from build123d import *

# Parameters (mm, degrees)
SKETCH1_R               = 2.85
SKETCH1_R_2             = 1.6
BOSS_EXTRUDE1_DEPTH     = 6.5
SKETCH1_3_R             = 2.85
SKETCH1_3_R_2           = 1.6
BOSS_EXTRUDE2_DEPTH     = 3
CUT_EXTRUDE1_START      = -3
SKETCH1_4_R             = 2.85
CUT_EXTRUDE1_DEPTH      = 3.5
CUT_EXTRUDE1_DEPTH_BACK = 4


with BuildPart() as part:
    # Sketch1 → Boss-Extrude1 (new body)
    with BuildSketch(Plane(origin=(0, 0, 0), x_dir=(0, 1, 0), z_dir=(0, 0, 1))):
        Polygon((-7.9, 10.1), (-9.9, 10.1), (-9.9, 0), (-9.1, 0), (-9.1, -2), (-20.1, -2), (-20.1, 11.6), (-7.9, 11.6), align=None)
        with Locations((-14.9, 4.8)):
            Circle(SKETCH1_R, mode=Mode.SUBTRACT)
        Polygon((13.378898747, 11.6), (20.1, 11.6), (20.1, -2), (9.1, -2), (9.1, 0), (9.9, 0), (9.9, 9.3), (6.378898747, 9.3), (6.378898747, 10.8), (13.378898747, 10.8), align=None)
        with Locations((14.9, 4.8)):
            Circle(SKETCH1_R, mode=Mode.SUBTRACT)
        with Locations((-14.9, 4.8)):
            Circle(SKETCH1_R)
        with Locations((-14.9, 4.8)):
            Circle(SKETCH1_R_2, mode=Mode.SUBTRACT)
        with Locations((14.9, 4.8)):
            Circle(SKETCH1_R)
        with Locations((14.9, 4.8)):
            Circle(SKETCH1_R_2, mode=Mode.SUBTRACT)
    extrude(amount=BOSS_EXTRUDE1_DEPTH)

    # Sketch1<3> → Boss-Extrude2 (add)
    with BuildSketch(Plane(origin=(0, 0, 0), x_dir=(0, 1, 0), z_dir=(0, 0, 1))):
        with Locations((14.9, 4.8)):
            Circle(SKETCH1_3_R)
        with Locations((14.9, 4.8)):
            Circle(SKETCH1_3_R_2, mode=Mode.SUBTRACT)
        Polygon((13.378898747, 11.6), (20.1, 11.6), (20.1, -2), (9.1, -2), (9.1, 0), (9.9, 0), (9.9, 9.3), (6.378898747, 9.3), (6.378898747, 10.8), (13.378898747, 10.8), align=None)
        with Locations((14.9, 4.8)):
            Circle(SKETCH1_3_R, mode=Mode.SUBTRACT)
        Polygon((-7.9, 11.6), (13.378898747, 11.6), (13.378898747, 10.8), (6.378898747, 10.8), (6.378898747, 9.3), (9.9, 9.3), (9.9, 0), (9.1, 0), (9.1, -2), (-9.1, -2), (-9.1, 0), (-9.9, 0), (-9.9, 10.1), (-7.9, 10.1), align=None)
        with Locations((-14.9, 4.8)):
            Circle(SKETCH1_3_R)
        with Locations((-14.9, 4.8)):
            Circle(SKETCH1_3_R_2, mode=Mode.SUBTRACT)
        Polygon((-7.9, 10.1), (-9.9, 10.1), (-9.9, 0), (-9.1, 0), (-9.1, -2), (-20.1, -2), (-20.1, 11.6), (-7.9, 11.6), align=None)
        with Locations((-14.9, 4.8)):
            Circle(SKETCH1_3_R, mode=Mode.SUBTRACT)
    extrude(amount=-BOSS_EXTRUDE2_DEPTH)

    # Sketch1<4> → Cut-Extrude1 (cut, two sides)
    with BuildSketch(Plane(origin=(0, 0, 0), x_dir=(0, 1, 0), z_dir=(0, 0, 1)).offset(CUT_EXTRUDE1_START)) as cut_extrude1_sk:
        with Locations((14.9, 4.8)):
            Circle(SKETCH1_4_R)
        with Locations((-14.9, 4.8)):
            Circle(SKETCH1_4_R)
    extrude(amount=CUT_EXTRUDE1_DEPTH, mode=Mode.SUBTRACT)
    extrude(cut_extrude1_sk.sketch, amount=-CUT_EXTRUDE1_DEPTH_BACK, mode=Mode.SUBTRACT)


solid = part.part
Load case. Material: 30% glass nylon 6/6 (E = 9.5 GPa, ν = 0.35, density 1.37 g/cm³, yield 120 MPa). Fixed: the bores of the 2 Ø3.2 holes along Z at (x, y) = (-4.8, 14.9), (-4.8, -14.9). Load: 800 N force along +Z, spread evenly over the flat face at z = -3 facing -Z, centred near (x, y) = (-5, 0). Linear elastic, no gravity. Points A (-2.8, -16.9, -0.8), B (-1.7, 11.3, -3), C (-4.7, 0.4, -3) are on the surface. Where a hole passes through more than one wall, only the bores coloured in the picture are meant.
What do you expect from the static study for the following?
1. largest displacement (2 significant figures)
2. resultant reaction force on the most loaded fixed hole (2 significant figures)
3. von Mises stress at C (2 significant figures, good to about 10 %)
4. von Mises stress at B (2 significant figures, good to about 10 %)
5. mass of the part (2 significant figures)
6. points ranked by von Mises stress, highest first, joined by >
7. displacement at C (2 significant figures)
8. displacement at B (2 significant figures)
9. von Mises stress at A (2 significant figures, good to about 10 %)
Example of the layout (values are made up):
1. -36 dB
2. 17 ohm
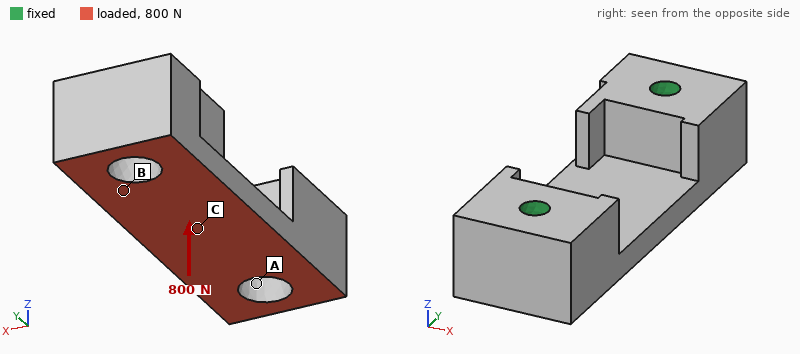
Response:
1. 72 µm
2. 450 N
3. 22 MPa
4. 12 MPa
5. 4.4 g
6. C > B > A
7. 60 µm
8. 13 µm
9. 4.5 MPa
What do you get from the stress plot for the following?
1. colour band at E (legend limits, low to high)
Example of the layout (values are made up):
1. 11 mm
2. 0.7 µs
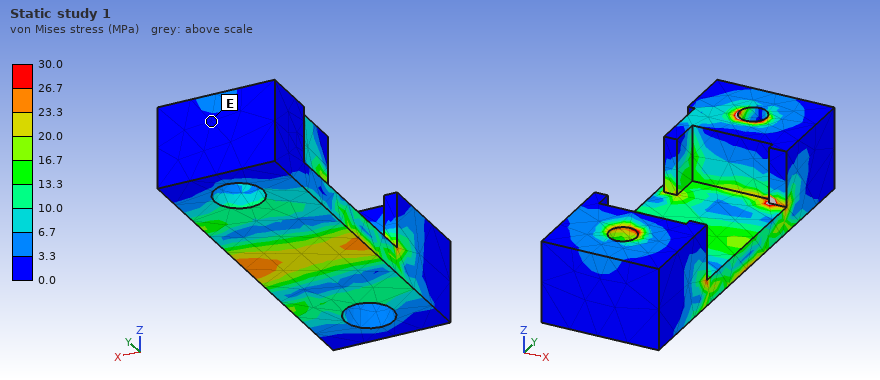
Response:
1. 0.0 to 3.3 MPa
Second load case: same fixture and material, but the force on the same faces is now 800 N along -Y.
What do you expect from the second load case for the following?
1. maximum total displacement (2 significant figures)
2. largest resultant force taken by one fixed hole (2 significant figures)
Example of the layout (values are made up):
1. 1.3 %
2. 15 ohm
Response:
1. 22 µm
2. 410 N
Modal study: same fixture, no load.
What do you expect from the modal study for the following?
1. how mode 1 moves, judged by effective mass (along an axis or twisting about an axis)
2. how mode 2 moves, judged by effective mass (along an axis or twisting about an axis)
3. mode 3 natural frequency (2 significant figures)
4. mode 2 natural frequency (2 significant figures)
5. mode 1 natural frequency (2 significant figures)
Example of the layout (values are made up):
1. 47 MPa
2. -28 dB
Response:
1. along Z
2. along X
3. 20 kHz
4. 15 kHz
5. 14 kHz
